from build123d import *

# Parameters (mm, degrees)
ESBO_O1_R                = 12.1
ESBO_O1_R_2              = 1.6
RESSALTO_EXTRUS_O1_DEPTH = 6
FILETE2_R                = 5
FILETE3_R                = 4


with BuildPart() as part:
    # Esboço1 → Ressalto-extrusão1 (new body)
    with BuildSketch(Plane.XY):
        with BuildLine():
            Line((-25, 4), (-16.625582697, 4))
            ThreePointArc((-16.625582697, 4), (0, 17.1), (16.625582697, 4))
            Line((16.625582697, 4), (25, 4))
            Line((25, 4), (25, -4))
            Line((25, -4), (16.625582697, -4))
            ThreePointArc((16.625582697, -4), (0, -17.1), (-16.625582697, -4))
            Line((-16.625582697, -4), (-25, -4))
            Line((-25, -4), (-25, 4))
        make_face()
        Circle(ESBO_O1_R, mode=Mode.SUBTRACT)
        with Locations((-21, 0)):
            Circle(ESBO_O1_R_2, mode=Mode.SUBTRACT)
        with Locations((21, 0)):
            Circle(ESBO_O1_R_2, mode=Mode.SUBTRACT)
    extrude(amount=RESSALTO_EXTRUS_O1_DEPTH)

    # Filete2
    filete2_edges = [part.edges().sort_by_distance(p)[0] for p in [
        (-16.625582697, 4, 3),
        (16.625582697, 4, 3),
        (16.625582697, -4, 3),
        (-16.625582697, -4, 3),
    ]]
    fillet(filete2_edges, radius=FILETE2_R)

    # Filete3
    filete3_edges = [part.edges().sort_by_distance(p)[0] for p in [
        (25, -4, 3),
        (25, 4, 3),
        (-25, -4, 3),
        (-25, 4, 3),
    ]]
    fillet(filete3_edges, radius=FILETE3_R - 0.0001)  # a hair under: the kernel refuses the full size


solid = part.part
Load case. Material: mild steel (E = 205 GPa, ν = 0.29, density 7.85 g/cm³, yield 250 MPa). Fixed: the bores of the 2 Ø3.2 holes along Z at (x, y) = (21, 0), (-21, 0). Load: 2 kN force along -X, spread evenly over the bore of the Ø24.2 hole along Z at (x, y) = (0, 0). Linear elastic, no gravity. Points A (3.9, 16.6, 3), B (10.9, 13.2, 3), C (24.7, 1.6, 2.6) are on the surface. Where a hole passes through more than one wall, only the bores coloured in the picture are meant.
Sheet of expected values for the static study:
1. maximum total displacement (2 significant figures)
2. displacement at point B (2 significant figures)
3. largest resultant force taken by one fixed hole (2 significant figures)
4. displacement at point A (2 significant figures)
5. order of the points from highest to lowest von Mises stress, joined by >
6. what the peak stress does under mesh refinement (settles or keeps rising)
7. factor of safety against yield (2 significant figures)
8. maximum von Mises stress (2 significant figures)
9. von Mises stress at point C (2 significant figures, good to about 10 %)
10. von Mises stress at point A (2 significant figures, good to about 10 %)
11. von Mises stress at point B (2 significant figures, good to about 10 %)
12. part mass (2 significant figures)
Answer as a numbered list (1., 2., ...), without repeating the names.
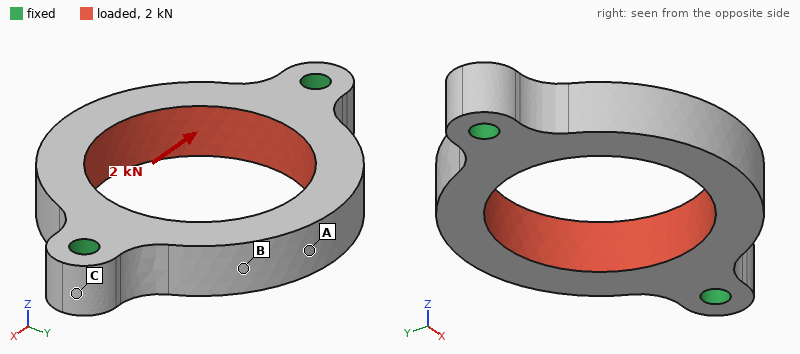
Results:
1. 3.8 µm
2. 3.6 µm
3. 1.0 kN
4. 2.9 µm
5. B > A > C
6. settles
7. 4.6
8. 54 MPa
9. 4.9 MPa
10. 11 MPa
11. 17 MPa
12. 27 g
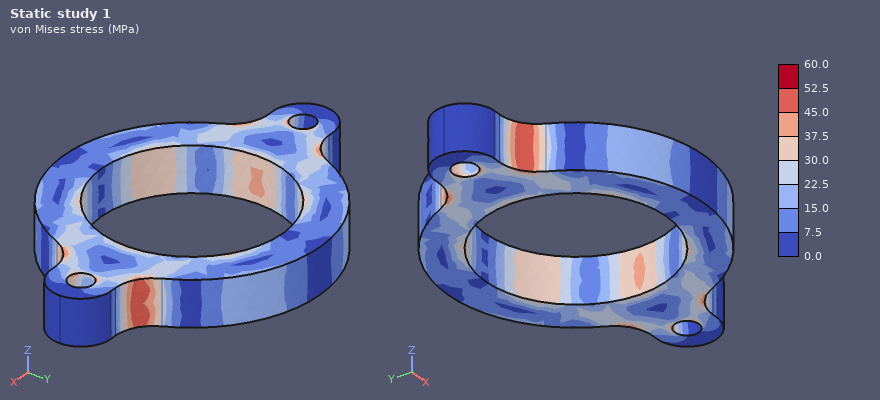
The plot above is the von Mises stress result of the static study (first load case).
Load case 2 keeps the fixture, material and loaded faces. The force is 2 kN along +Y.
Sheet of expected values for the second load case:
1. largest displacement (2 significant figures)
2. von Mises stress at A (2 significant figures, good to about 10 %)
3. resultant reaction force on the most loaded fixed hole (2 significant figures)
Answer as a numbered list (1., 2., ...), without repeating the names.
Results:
1. 3.2 µm
2. 10 MPa
3. 1.0 kN
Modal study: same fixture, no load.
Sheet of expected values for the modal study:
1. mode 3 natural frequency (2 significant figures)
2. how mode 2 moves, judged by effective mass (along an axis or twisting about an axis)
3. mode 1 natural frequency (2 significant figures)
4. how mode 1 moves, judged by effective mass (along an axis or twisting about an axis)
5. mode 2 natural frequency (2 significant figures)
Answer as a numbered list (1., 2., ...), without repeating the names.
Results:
1. 20 kHz
2. along Z
3. 8700 Hz
4. twisting about X
5. 11 kHz
